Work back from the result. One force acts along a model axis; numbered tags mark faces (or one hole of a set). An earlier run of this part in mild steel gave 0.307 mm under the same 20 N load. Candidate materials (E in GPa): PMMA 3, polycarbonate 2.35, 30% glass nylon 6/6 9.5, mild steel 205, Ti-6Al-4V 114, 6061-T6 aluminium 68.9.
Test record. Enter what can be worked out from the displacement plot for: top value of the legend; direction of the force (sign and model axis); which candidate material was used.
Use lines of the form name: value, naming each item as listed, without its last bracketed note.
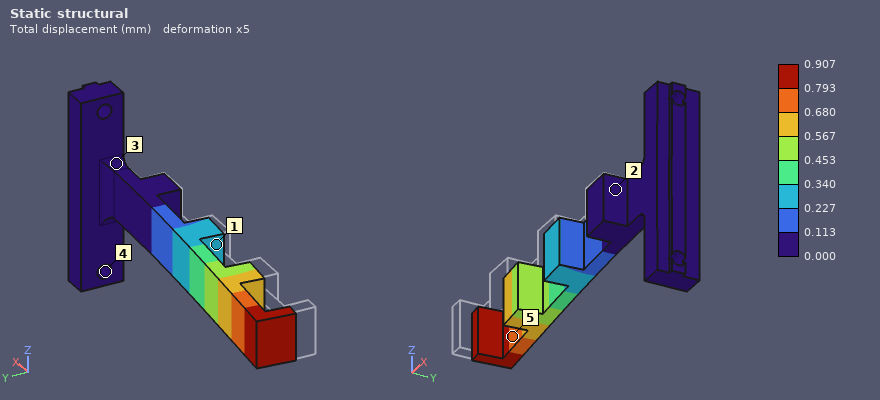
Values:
top value of the legend: 0.907 mm
direction of the force: +Y
which candidate material was used: 6061-T6 aluminium
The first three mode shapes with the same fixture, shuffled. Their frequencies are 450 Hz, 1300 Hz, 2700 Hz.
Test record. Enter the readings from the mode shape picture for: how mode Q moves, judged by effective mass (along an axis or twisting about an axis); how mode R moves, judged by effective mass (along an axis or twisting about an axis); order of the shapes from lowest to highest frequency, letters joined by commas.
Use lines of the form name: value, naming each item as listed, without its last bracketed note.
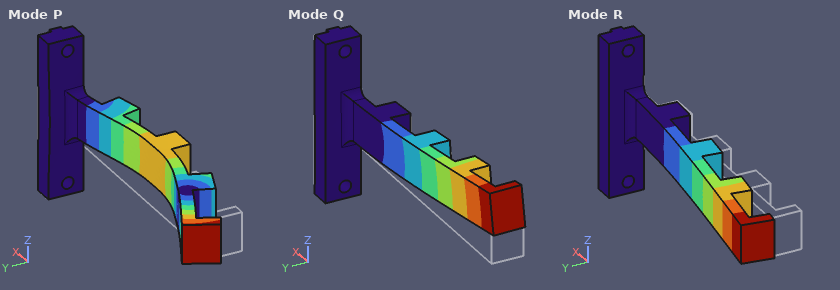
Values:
how mode Q moves, judged by effective mass: along Z
how mode R moves, judged by effective mass: along Y
order of the shapes from lowest to highest frequency, letters joined by commas: R, Q, P
